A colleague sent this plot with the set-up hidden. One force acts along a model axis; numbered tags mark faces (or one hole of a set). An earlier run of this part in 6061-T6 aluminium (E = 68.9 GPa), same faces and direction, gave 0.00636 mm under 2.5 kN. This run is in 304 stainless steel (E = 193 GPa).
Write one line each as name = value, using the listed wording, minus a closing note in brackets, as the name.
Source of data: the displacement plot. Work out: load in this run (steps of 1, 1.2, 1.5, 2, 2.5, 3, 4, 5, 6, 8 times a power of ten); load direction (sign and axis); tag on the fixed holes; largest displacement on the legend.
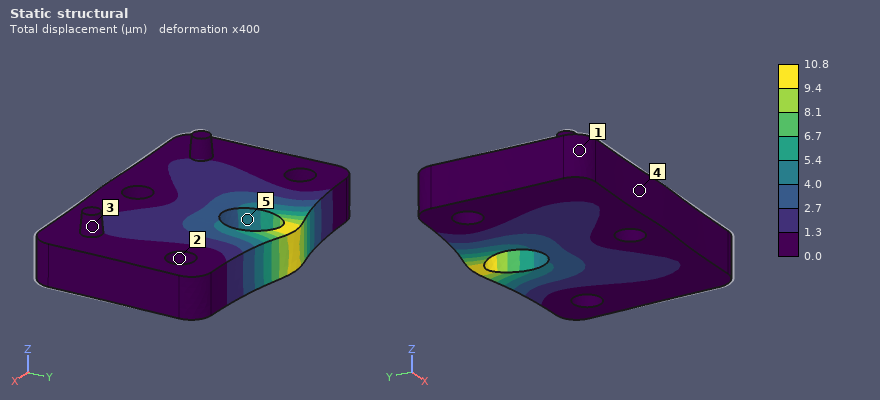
load in this run = 12 kN
load direction = +Y
tag on the fixed holes = 2
largest displacement on the legend = 10.8 µm
